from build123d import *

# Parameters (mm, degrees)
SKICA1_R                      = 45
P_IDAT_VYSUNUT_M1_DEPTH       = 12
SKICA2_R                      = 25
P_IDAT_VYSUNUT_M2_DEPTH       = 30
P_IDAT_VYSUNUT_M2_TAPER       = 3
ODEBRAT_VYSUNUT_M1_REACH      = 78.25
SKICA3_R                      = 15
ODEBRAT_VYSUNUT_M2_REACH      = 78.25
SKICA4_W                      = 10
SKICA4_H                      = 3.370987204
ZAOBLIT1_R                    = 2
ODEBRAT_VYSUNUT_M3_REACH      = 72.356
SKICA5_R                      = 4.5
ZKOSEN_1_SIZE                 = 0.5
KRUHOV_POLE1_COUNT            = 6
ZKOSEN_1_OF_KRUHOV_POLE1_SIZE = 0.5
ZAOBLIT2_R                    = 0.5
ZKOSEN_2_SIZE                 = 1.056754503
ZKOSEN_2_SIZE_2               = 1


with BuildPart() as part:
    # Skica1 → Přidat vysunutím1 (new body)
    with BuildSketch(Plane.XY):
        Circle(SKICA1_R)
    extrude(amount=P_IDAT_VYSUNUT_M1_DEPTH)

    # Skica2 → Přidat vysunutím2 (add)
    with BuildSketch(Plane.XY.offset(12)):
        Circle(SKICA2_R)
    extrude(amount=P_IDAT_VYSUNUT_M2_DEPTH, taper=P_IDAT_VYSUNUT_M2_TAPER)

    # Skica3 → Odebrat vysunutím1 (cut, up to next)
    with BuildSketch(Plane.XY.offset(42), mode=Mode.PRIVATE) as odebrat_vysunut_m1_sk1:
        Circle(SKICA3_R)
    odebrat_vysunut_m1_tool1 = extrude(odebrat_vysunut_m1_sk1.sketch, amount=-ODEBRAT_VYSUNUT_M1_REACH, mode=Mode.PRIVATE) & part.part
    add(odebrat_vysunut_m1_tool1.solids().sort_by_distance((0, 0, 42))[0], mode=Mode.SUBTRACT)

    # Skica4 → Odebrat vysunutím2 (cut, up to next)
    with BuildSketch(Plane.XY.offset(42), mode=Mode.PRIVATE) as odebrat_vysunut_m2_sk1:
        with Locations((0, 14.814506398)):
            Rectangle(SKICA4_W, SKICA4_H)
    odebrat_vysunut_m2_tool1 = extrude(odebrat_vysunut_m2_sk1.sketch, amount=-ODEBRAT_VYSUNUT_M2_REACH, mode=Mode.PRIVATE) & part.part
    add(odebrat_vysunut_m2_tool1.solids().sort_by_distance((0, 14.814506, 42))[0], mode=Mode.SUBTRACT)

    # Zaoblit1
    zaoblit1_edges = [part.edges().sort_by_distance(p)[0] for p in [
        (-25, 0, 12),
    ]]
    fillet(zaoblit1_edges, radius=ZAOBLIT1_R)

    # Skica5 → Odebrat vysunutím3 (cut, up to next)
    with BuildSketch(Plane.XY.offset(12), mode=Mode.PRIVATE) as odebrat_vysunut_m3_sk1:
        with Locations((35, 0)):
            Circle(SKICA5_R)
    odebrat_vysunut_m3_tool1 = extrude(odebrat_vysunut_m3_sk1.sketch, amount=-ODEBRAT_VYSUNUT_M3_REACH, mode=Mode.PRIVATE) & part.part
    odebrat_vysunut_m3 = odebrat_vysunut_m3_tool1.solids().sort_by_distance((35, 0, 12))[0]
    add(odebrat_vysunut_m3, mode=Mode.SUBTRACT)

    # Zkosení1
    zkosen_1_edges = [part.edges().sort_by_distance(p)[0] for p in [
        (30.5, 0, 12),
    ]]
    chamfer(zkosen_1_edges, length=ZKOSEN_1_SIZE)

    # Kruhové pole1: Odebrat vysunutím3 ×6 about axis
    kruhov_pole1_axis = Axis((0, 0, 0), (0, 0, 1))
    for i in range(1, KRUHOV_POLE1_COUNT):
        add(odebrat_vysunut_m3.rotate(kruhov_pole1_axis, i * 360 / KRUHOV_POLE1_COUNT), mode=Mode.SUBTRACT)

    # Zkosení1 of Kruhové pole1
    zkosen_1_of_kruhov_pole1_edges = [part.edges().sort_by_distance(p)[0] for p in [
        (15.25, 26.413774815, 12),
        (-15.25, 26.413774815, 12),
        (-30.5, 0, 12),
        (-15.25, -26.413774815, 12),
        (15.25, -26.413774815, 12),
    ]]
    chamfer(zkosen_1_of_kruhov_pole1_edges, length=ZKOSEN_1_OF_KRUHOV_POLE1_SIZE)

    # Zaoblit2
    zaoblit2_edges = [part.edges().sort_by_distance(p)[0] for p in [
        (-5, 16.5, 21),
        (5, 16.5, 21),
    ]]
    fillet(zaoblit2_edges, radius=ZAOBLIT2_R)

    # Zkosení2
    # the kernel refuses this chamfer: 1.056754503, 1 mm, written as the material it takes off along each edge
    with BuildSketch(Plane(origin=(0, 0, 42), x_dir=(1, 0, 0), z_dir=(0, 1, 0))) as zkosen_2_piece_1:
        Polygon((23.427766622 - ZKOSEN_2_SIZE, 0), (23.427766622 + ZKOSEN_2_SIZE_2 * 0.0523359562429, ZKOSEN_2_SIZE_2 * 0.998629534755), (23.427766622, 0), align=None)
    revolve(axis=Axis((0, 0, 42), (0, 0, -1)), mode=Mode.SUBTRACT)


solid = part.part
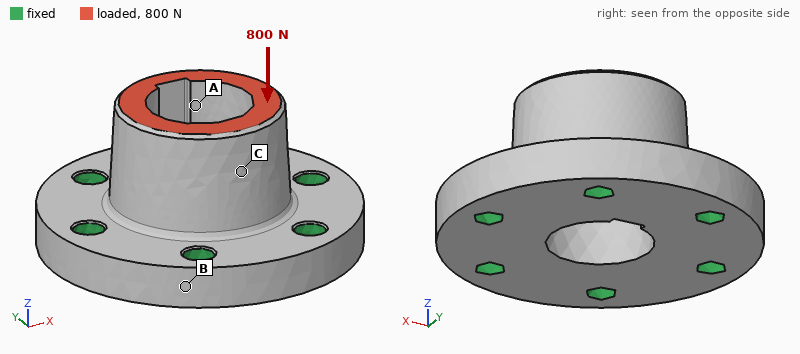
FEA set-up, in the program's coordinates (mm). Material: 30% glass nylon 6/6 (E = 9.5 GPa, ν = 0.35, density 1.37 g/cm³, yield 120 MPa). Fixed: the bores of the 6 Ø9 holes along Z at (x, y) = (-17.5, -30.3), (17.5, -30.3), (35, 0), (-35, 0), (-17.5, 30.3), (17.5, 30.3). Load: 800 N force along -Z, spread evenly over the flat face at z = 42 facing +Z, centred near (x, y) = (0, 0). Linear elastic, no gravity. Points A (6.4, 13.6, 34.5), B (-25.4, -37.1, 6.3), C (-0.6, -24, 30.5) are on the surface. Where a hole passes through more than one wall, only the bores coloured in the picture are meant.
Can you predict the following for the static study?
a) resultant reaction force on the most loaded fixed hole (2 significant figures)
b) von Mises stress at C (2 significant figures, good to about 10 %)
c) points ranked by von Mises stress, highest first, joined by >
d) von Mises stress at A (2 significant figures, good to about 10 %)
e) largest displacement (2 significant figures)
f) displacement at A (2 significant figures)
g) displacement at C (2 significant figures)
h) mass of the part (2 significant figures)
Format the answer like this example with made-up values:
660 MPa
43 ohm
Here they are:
150 N
0.55 MPa
A > C > B
1.0 MPa
4.8 µm
4.0 µm
3.8 µm
130 g
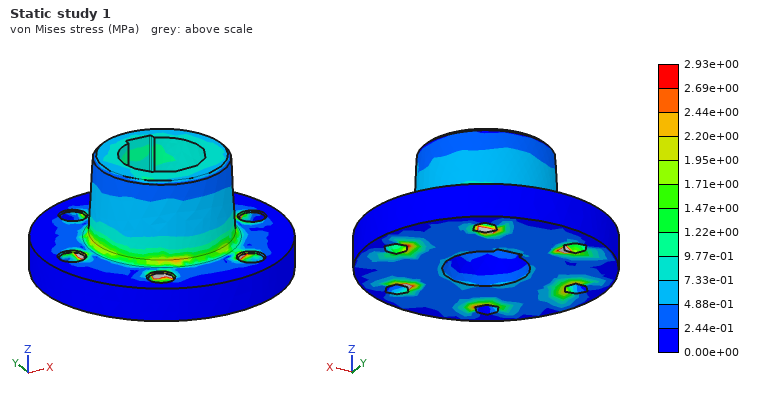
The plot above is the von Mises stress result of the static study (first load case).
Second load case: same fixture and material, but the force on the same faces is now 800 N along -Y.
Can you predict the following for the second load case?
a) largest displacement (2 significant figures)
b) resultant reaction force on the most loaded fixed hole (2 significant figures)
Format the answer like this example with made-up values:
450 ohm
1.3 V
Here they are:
26 µm
330 N
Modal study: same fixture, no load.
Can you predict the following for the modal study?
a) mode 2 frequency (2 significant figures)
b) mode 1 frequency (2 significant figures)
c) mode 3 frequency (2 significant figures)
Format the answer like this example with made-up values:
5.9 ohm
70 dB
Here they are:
7500 Hz
7500 Hz
9400 Hz
